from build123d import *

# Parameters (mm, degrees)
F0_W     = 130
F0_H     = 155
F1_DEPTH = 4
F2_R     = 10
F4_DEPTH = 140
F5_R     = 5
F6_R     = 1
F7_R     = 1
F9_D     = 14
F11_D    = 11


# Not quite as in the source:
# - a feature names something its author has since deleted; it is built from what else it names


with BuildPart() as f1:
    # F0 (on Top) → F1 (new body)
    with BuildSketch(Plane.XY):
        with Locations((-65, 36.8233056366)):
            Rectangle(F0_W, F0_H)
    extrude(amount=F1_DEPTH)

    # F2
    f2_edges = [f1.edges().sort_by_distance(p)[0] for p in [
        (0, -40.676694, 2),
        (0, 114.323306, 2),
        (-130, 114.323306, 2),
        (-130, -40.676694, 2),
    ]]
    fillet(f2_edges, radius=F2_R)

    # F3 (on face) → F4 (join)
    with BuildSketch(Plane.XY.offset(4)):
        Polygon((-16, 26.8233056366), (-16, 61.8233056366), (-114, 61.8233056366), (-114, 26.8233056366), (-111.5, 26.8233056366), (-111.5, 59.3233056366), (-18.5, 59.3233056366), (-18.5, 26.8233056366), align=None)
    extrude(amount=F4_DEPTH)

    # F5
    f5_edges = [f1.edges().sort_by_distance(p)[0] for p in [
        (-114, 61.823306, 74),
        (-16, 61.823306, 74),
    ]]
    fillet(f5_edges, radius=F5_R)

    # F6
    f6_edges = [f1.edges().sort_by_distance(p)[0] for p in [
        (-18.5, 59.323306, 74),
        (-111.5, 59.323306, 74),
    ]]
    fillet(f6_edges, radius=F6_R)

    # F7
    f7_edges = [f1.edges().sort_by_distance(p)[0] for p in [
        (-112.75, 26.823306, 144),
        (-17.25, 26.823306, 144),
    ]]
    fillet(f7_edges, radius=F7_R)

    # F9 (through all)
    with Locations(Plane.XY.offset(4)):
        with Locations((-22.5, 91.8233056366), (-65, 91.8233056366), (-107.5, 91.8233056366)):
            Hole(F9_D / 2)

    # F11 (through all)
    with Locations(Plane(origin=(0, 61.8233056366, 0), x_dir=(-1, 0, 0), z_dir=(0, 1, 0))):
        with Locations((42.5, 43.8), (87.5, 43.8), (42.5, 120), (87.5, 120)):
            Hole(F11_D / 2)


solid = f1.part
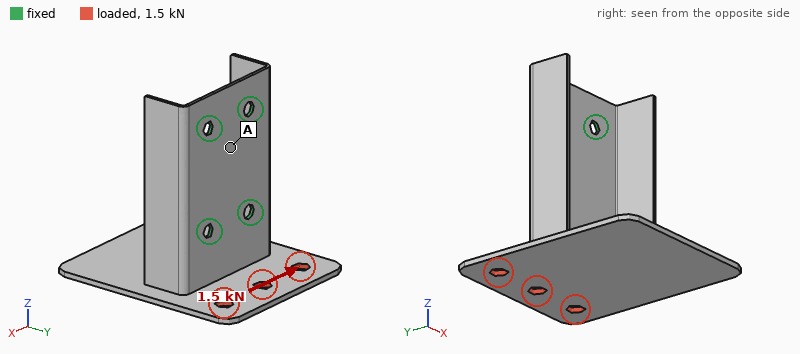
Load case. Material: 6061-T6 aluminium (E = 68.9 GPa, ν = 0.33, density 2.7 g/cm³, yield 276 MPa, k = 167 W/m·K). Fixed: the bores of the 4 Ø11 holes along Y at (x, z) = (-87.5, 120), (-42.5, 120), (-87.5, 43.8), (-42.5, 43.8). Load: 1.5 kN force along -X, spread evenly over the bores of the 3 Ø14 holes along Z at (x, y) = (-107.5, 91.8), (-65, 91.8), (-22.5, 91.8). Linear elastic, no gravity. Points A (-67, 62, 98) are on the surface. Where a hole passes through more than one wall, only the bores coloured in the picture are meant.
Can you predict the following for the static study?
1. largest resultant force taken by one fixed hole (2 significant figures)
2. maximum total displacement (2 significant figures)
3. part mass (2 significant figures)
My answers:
1.3 kN
1.4 mm
360 g
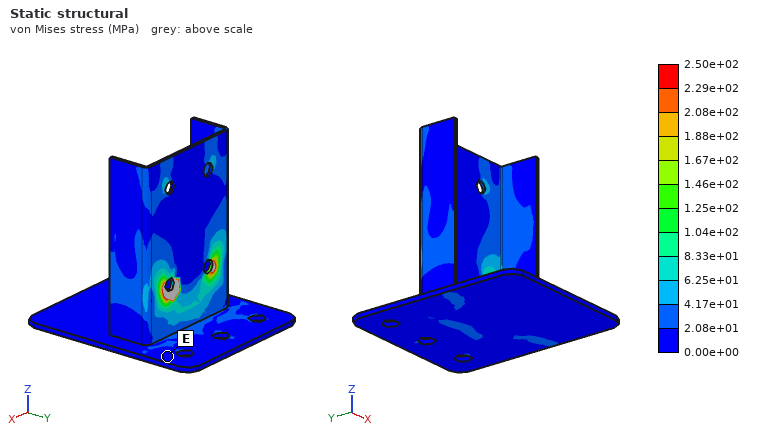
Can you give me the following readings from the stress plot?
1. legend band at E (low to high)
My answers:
0.00e+00 to 2.08e+01 MPa
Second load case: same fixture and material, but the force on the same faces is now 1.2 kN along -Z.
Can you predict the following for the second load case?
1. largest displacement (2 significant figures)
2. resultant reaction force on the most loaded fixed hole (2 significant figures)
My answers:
1.0 mm
850 N
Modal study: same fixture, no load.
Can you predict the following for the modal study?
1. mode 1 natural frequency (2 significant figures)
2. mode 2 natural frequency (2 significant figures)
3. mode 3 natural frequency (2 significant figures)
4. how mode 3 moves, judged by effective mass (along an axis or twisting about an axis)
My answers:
330 Hz
380 Hz
620 Hz
along Y
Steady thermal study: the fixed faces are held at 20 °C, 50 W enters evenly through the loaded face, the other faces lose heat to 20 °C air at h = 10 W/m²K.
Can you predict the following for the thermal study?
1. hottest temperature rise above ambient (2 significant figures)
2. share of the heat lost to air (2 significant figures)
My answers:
50 K
31 %
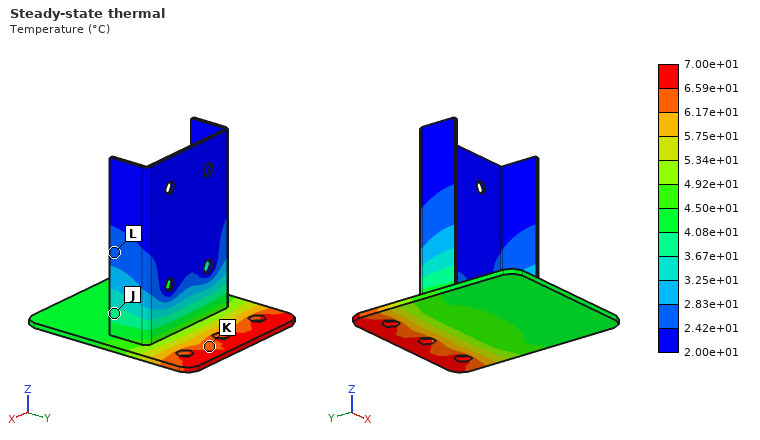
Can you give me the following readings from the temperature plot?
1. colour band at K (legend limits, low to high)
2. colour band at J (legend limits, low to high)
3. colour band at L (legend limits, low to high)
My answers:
6.17e+01 to 6.59e+01 °C
3.67e+01 to 4.08e+01 °C
2.42e+01 to 2.83e+01 °C
